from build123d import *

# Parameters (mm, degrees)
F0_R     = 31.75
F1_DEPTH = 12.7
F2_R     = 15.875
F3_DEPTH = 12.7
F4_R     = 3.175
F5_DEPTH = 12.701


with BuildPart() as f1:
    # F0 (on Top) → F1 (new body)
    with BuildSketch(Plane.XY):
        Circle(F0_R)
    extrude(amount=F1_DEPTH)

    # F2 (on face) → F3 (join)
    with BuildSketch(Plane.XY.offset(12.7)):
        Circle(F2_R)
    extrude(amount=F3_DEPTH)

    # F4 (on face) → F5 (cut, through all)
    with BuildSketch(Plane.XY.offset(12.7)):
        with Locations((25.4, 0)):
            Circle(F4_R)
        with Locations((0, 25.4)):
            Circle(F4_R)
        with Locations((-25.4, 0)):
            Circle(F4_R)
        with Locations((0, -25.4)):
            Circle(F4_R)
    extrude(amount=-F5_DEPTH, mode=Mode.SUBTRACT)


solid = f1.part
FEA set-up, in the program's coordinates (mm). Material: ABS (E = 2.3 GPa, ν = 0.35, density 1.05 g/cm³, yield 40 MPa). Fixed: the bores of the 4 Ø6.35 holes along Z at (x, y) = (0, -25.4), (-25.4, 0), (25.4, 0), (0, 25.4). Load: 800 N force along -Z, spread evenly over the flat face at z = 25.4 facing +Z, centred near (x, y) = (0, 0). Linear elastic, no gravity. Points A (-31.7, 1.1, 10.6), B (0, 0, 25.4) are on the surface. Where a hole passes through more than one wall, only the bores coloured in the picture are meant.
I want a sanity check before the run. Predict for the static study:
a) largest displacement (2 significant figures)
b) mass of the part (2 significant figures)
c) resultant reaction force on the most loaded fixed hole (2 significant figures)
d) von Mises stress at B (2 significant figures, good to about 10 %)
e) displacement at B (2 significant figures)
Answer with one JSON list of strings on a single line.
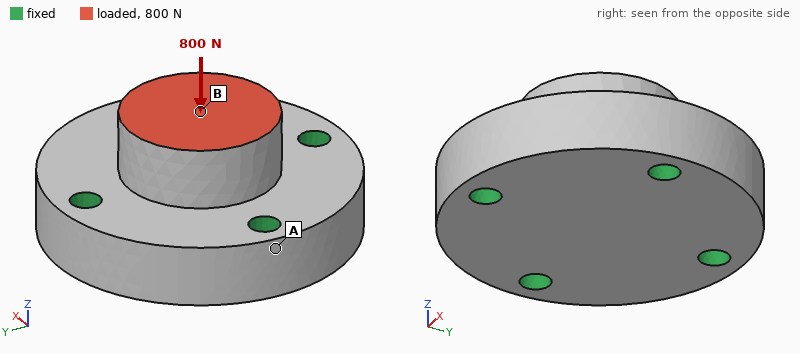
["22 µm", "51 g", "210 N", "0.73 MPa", "22 µm"]
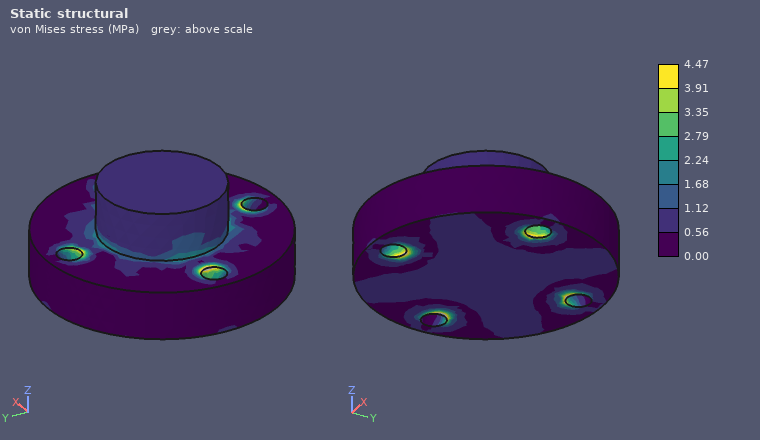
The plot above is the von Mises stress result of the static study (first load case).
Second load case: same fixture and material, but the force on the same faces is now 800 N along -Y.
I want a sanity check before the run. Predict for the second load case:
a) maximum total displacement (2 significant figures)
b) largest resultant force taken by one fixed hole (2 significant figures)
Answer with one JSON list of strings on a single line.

["62 µm", "410 N"]
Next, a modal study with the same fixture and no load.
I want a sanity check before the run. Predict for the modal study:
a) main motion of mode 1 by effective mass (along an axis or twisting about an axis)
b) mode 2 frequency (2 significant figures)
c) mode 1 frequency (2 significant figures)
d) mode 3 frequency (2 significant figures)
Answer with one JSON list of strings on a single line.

["along Z", "7100 Hz", "6700 Hz", "7100 Hz"]
